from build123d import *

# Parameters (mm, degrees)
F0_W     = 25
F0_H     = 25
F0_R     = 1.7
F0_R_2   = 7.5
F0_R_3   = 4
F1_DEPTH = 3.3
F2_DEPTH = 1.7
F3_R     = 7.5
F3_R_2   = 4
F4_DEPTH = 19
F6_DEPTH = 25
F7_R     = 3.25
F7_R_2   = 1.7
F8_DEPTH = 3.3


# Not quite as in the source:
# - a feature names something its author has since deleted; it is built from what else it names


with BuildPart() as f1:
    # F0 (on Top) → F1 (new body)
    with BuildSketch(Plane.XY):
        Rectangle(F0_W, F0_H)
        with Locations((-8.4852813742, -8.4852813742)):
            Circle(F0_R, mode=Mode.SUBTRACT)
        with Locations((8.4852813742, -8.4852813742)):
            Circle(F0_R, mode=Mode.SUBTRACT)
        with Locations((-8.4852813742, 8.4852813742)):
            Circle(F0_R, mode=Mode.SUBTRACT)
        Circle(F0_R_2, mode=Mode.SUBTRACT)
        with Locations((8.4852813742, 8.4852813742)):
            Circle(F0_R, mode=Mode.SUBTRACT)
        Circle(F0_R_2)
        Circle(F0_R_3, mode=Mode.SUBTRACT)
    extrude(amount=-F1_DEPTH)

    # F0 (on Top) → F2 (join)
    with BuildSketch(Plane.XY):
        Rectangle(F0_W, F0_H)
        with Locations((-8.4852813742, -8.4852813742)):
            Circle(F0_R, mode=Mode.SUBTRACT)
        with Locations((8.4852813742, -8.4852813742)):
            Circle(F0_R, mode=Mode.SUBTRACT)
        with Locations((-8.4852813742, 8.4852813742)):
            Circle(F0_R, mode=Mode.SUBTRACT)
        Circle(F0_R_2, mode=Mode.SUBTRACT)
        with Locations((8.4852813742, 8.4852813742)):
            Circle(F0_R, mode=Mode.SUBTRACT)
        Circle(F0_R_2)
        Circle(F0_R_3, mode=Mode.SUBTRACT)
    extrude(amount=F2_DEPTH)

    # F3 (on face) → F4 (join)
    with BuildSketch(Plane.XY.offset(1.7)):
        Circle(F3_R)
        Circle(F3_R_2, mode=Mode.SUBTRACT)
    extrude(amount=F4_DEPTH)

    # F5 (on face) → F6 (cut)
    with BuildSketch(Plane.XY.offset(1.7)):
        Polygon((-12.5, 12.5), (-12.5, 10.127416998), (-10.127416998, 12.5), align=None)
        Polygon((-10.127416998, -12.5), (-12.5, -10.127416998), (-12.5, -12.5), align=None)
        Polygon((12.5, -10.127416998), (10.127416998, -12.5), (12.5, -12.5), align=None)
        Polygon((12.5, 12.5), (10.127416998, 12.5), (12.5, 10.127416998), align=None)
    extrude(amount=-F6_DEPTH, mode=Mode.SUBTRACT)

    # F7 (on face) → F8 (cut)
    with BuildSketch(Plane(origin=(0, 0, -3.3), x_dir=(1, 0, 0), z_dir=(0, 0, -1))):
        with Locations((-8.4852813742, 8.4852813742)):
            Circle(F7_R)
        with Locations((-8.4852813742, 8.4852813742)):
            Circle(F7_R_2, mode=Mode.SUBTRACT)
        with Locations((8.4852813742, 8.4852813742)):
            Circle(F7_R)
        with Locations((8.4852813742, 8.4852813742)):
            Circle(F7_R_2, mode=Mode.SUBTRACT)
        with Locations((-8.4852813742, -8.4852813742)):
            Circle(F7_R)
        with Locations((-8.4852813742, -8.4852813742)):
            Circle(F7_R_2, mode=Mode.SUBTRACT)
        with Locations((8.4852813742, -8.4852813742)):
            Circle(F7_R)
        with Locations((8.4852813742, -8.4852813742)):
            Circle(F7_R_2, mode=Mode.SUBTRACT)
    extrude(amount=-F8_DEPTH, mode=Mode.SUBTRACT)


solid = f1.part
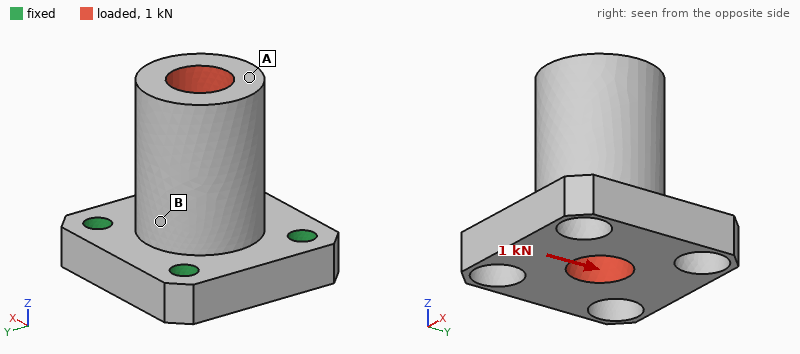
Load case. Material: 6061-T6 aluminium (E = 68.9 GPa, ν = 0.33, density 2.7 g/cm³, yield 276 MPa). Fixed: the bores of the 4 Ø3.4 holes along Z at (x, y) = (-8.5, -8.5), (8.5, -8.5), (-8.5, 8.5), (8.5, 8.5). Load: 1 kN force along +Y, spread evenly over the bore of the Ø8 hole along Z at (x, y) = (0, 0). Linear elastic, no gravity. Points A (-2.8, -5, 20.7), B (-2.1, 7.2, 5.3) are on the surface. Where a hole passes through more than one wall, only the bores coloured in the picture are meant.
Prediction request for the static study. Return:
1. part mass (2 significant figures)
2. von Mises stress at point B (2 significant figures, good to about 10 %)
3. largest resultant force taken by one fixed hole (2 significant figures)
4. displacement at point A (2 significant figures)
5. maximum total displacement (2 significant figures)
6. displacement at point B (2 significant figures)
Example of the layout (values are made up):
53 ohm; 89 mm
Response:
13 g; 15 MPa; 350 N; 22 µm; 23 µm; 8.2 µm
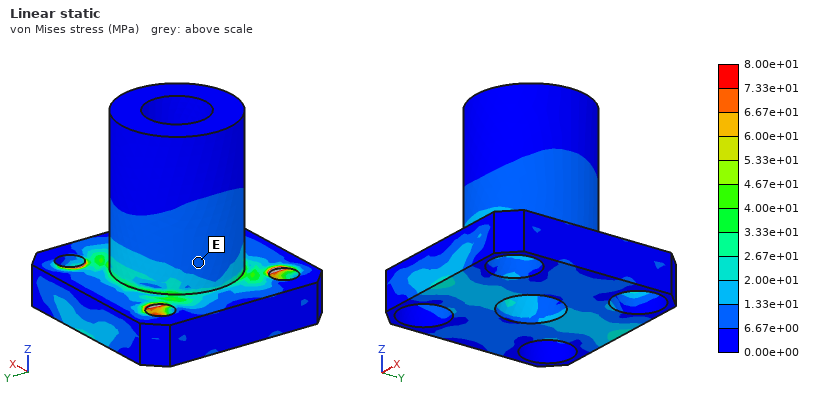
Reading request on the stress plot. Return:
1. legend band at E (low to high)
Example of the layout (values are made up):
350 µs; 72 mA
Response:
6.67e+00 to 1.33e+01 MPa
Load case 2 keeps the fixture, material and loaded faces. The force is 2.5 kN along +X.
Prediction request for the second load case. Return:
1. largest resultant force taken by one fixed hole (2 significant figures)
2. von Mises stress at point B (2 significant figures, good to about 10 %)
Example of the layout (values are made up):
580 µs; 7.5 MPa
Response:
870 N; 26 MPa
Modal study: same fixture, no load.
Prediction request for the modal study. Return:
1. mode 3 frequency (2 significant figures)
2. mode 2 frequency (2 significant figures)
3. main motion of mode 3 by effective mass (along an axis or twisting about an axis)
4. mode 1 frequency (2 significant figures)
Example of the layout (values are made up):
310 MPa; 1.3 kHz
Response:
24 kHz; 14 kHz; along Z; 14 kHz
